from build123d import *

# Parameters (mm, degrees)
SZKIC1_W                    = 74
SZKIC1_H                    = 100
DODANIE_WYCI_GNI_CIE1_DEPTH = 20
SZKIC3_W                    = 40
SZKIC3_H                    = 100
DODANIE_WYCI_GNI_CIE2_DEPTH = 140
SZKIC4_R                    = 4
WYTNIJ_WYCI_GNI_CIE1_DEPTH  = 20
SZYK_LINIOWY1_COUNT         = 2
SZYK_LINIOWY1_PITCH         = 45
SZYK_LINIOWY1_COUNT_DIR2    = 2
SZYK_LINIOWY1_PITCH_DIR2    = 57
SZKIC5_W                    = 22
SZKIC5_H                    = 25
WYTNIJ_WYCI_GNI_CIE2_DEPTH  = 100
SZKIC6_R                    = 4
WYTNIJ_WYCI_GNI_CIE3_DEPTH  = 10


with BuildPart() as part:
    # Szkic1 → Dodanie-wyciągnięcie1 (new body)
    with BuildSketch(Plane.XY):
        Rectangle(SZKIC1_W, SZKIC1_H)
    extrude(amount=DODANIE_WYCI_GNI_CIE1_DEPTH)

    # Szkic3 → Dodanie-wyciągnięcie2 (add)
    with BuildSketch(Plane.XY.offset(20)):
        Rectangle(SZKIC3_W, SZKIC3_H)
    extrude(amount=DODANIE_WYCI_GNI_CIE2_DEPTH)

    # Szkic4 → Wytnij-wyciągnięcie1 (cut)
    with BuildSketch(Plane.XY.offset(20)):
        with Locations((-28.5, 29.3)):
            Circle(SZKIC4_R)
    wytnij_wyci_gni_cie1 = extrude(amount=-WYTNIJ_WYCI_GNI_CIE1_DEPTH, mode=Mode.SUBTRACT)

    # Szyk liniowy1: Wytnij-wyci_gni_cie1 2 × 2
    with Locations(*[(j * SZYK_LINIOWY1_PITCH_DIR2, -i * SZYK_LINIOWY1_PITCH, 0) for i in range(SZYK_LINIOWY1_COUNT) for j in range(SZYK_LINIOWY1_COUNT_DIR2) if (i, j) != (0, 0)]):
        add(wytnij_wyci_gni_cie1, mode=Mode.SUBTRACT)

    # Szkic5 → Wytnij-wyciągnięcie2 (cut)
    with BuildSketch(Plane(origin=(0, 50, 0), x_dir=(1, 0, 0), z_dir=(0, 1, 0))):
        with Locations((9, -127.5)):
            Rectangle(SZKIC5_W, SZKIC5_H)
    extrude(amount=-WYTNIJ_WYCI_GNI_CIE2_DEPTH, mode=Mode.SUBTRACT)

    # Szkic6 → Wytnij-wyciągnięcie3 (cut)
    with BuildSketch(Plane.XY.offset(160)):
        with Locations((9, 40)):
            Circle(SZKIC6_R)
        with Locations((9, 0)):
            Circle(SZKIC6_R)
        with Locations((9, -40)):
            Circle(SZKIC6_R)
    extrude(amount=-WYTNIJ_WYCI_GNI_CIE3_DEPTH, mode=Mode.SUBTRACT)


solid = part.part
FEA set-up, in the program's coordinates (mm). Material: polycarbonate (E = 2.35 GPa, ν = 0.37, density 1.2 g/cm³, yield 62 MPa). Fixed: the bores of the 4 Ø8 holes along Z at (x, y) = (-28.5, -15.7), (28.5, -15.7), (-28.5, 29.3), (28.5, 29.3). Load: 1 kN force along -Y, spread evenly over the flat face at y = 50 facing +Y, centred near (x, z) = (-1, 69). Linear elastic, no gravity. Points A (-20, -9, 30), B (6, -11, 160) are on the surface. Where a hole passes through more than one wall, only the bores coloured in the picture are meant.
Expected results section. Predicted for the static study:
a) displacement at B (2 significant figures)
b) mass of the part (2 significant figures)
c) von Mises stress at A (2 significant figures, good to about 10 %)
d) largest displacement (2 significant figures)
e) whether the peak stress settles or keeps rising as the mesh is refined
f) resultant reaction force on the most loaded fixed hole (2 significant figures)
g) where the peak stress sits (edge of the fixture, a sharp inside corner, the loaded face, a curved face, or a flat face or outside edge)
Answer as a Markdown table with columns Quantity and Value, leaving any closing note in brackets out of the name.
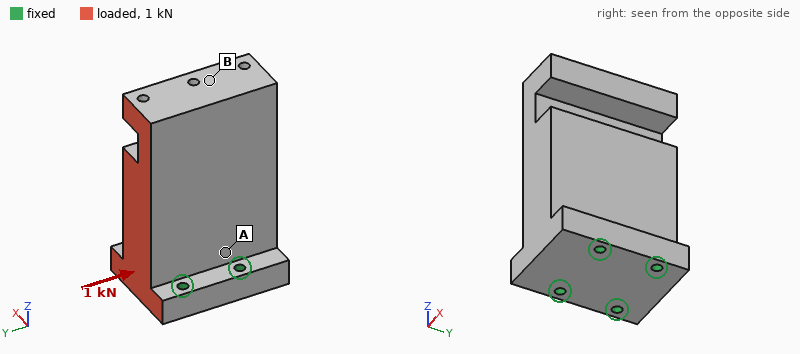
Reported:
| Quantity | Value |
|---|---|
| displacement at B | 0.19 mm |
| mass of the part | 780 g |
| von Mises stress at A | 0.84 MPa |
| largest displacement | 0.20 mm |
| whether the peak stress settles or keeps rising as the mesh is refined | keeps rising |
| resultant reaction force on the most loaded fixed hole | 570 N |
| where the peak stress sits | edge of the fixture |
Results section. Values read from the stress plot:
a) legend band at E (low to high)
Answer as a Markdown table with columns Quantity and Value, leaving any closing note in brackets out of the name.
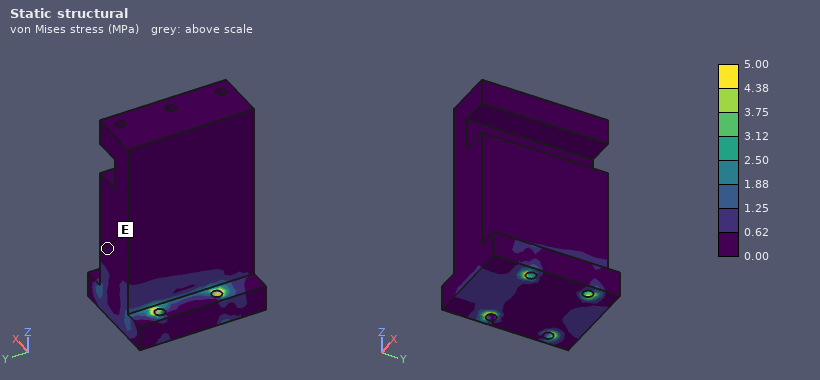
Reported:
| Quantity | Value |
|---|---|
| legend band at E | 0.00 to 0.62 MPa |
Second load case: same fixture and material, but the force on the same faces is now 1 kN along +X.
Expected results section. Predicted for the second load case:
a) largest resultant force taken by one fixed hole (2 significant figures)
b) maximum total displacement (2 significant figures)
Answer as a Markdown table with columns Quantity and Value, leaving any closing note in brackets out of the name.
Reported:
| Quantity | Value |
|---|---|
| largest resultant force taken by one fixed hole | 800 N |
| maximum total displacement | 0.50 mm |
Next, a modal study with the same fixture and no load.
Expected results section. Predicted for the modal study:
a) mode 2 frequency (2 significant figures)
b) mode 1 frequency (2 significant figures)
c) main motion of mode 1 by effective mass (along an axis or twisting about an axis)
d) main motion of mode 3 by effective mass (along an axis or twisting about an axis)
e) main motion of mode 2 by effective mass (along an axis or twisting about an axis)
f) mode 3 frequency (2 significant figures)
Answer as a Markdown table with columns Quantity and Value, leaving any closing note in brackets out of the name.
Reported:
| Quantity | Value |
|---|---|
| mode 2 frequency | 500 Hz |
| mode 1 frequency | 380 Hz |
| main motion of mode 1 by effective mass | along X |
| main motion of mode 3 by effective mass | twisting about Z |
| main motion of mode 2 by effective mass | along Y |
| mode 3 frequency | 930 Hz |
